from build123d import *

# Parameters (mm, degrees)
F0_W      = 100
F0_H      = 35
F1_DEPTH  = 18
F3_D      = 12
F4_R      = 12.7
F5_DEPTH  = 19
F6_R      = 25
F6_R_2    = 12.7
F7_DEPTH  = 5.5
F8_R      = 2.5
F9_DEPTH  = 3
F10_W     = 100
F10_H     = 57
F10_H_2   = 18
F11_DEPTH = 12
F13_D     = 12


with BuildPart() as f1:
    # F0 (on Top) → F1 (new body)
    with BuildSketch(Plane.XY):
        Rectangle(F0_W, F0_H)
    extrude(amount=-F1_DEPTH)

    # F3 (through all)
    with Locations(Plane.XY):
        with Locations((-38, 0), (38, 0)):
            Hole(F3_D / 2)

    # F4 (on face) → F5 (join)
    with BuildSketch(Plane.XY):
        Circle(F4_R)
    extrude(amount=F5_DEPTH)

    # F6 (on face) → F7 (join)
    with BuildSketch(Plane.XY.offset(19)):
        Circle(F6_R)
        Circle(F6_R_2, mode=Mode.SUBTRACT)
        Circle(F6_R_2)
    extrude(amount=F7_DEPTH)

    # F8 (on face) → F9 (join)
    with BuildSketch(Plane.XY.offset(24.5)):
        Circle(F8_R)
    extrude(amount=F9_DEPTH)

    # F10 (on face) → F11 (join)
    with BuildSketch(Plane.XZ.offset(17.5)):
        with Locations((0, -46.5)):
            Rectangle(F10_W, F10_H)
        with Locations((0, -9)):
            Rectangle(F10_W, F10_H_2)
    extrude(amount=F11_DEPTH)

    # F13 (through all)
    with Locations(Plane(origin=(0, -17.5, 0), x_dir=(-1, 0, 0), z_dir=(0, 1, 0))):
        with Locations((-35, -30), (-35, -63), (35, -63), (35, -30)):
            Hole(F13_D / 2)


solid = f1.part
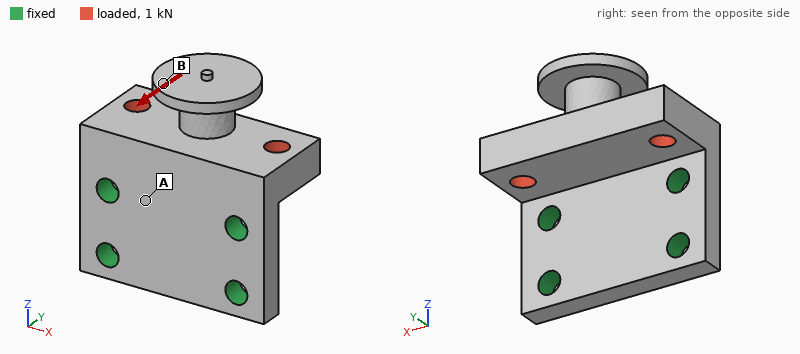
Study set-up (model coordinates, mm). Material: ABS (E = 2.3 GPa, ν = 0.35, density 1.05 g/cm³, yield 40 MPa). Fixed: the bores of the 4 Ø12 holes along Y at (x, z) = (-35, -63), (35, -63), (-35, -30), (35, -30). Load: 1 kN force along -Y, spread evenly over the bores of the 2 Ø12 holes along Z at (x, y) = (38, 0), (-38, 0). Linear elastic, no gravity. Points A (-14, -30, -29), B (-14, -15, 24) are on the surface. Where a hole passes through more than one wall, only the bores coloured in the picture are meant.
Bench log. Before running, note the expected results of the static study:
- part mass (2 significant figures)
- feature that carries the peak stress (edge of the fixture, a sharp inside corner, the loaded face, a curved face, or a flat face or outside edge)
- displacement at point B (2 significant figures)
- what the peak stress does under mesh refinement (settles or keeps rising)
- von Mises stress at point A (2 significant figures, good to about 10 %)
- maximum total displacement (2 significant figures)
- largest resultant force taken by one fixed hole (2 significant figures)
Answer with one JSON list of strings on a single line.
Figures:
["170 g", "edge of the fixture", "0.30 mm", "keeps rising", "2.4 MPa", "0.41 mm", "560 N"]
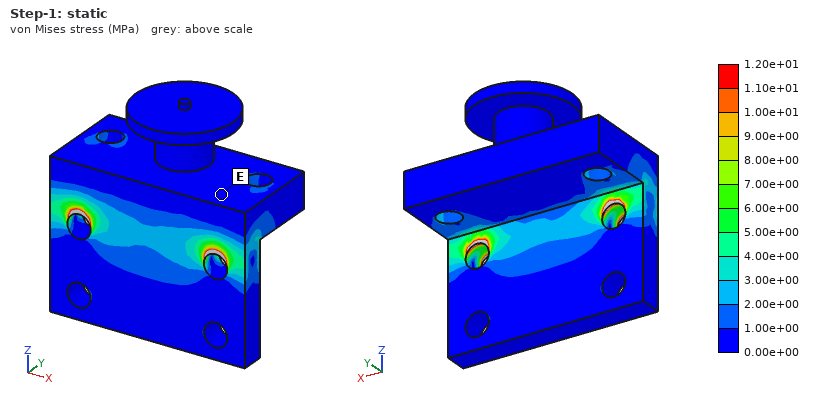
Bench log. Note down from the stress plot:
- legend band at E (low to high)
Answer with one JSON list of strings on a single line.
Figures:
["0.00e+00 to 1.00e+00 MPa"]
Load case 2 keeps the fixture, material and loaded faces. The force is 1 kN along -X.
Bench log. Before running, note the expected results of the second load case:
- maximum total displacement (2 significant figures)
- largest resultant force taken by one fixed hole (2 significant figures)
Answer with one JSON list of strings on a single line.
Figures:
["0.10 mm", "610 N"]
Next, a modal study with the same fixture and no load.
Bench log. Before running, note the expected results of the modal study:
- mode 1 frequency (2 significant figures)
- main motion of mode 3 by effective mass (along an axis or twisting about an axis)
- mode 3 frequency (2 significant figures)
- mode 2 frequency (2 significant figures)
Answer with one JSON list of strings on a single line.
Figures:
["660 Hz", "along X", "2000 Hz", "1700 Hz"]
